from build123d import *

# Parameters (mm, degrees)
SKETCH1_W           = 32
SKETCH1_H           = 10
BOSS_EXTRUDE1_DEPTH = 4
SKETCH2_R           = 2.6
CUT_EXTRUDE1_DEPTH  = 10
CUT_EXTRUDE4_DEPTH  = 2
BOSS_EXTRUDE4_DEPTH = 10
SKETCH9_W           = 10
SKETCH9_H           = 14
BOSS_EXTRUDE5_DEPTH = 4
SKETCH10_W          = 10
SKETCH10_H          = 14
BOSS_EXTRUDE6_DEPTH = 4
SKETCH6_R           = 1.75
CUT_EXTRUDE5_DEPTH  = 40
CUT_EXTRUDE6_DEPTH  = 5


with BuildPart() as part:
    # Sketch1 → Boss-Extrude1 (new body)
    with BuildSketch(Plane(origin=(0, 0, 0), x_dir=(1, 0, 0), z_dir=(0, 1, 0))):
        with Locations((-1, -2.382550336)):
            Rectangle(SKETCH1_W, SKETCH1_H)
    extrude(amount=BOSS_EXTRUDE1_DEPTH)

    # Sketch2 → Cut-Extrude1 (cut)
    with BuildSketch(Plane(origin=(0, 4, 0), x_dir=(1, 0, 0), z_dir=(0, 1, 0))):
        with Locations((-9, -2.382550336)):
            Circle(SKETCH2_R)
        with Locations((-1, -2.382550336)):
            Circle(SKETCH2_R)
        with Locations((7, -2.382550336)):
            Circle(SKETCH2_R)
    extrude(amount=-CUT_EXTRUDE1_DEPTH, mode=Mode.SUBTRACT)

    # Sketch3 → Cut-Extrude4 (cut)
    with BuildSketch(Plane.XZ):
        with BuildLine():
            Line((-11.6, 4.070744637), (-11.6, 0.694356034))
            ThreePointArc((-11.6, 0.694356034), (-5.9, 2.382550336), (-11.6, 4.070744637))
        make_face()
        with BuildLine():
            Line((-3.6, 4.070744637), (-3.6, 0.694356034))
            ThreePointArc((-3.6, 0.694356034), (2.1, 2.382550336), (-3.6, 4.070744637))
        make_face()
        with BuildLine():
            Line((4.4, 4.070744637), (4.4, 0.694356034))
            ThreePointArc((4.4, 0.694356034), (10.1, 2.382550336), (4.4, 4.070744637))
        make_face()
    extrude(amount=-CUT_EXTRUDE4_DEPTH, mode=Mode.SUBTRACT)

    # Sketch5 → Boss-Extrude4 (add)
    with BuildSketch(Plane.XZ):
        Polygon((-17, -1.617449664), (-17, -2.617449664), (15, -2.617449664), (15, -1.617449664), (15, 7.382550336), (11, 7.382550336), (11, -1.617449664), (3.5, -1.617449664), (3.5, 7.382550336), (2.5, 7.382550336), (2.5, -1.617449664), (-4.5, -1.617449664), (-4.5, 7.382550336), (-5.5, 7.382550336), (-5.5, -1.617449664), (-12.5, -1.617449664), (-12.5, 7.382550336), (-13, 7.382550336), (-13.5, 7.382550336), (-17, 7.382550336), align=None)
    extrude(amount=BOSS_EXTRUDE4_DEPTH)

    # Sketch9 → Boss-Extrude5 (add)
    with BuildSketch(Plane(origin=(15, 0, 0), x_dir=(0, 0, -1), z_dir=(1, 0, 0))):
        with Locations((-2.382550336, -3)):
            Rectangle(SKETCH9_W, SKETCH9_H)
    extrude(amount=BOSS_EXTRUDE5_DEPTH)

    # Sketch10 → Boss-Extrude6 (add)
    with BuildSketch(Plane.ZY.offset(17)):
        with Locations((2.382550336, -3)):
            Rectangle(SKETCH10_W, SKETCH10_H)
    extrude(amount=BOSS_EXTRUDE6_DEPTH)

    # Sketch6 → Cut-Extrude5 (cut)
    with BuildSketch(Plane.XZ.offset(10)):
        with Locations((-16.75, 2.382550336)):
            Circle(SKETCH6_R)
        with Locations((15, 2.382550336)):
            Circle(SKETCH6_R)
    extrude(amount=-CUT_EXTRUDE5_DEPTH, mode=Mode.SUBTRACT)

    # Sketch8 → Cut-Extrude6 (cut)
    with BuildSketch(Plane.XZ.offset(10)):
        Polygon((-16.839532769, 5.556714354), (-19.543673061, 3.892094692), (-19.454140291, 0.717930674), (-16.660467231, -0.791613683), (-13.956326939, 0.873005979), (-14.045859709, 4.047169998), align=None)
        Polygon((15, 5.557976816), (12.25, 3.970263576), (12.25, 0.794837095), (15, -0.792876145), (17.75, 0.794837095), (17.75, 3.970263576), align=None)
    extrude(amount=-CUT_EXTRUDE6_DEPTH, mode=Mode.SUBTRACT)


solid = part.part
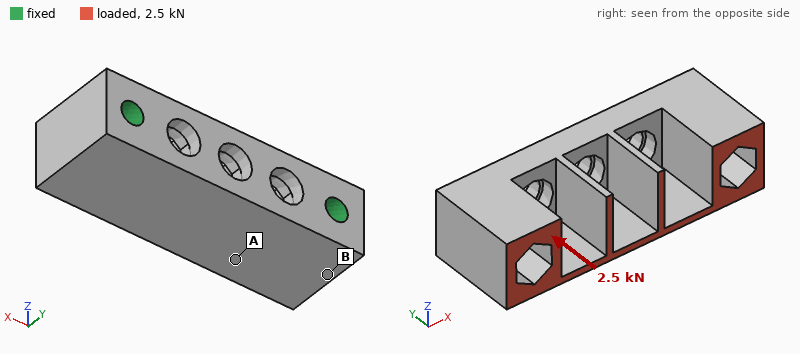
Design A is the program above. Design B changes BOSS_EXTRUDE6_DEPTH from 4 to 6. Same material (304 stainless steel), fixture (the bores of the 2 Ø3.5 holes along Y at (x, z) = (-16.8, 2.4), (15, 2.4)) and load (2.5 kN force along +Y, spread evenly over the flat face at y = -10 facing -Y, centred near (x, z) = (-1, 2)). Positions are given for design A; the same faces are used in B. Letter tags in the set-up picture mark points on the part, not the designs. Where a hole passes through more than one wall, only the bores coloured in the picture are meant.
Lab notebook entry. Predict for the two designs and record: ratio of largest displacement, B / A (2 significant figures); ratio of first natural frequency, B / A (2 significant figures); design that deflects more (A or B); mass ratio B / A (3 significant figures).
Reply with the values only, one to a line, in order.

0.88
1.00
A
1.10
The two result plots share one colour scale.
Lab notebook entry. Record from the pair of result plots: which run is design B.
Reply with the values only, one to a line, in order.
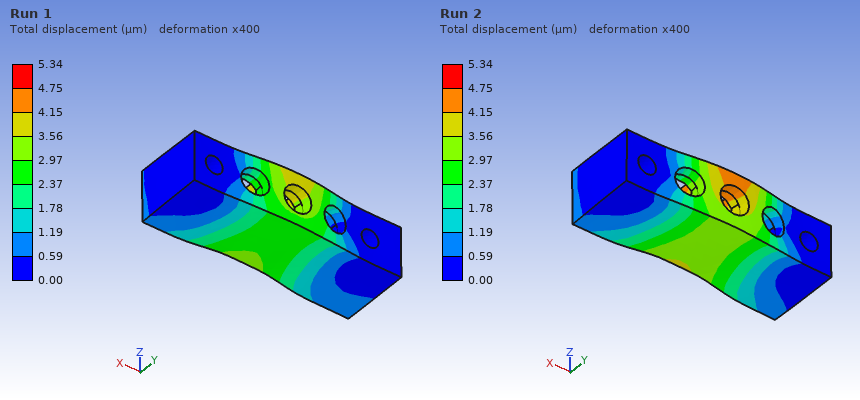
Run 1
